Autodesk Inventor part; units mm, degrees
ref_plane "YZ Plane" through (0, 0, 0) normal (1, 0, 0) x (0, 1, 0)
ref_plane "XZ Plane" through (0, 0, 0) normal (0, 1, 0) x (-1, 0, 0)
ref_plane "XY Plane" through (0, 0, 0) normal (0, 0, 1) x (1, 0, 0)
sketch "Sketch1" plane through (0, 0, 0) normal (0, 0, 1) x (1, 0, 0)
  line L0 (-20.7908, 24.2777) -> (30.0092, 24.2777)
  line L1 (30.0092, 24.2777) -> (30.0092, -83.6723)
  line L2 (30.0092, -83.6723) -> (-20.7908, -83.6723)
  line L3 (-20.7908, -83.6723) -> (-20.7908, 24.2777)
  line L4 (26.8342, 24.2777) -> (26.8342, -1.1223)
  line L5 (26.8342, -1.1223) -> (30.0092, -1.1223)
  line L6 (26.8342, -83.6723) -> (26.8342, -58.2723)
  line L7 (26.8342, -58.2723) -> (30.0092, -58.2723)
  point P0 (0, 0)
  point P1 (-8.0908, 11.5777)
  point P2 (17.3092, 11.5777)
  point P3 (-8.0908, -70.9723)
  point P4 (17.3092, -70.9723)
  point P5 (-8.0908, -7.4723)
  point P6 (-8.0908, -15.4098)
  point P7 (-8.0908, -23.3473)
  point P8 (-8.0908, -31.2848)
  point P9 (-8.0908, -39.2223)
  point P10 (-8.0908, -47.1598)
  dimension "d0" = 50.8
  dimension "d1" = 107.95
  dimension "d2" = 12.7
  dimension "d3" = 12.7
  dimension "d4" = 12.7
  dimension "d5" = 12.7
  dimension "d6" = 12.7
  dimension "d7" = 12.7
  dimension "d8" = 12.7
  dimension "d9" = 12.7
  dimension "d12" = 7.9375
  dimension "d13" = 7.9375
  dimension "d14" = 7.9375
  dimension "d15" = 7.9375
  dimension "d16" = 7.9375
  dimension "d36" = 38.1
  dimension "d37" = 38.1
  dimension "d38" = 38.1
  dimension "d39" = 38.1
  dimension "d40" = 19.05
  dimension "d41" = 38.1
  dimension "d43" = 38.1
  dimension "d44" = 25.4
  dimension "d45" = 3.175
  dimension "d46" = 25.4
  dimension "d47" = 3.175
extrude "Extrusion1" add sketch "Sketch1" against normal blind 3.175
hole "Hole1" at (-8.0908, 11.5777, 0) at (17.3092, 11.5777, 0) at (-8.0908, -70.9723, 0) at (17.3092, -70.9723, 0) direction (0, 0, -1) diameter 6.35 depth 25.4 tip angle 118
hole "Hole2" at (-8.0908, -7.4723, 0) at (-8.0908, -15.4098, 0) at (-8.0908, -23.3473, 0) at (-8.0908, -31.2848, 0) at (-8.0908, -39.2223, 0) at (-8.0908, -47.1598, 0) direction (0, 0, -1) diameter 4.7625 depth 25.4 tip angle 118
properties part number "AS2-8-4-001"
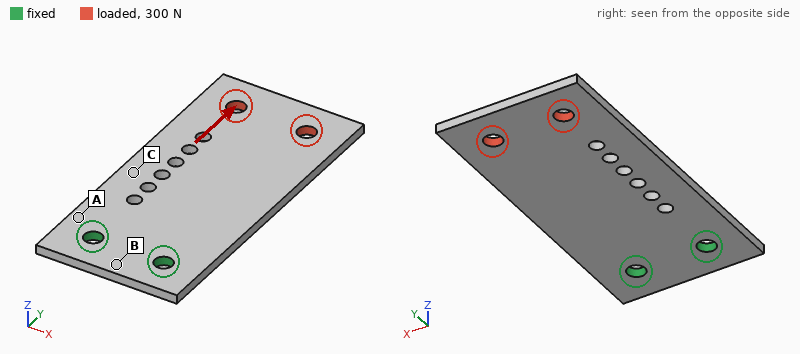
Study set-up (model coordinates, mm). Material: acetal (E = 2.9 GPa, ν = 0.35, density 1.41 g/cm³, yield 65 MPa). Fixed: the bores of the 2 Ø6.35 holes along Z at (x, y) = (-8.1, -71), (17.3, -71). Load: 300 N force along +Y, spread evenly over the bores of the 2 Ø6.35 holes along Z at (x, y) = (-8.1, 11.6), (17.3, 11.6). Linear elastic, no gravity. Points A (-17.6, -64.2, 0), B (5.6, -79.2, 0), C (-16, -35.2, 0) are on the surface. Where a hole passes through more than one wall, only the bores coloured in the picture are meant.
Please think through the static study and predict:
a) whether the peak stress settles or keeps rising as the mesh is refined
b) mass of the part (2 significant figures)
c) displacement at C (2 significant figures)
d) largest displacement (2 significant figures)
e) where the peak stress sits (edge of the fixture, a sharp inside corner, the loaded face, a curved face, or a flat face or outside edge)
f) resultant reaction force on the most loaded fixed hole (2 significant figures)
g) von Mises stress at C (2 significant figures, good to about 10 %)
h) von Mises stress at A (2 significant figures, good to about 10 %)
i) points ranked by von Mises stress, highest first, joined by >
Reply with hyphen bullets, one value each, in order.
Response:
- keeps rising
- 24 g
- 29 µm
- 69 µm
- edge of the fixture
- 150 N
- 2.2 MPa
- 1.3 MPa
- C > A > B
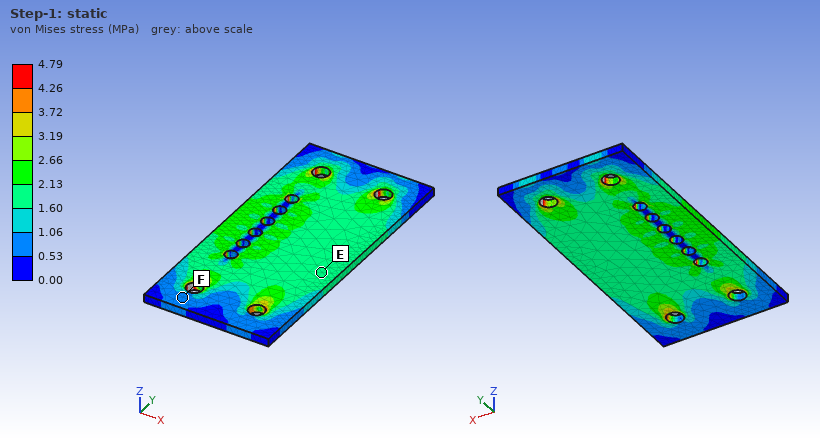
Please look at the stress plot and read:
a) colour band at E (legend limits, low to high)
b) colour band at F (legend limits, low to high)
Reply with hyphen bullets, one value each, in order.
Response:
- 1.60 to 2.13 MPa
- 0.53 to 1.06 MPa
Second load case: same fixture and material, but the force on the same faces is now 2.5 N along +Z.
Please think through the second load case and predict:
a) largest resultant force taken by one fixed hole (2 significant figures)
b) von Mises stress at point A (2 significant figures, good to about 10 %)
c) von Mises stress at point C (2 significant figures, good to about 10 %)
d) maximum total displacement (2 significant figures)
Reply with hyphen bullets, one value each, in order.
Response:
- 1.3 N
- 1.8 MPa
- 1.5 MPa
- 1.4 mm
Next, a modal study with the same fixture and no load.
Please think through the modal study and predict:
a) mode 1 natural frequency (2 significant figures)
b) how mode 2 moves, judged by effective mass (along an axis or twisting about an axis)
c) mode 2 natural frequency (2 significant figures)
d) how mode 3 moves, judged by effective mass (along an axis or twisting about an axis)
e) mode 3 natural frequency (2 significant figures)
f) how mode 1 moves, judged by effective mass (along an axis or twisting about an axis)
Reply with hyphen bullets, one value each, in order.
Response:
- 86 Hz
- twisting about Y
- 320 Hz
- along Z
- 520 Hz
- along Z
